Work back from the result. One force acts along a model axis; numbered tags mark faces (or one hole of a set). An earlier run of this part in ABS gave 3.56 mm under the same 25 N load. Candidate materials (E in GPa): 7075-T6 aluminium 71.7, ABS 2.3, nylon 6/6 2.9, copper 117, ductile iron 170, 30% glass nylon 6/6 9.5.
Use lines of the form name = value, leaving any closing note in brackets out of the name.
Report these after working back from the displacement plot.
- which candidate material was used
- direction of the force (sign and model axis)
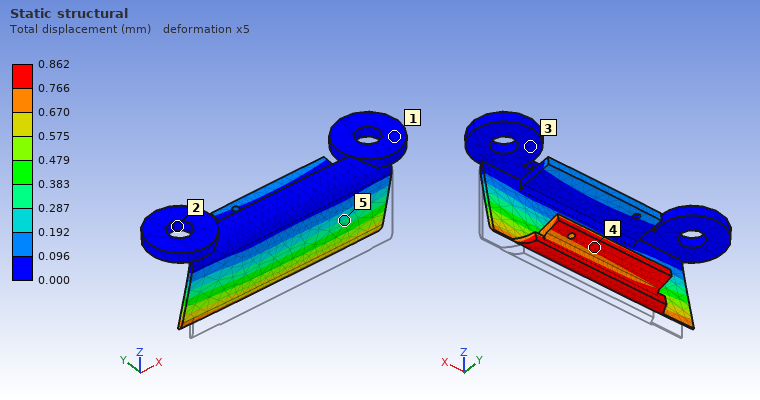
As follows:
which candidate material was used = 30% glass nylon 6/6
direction of the force = +Y
